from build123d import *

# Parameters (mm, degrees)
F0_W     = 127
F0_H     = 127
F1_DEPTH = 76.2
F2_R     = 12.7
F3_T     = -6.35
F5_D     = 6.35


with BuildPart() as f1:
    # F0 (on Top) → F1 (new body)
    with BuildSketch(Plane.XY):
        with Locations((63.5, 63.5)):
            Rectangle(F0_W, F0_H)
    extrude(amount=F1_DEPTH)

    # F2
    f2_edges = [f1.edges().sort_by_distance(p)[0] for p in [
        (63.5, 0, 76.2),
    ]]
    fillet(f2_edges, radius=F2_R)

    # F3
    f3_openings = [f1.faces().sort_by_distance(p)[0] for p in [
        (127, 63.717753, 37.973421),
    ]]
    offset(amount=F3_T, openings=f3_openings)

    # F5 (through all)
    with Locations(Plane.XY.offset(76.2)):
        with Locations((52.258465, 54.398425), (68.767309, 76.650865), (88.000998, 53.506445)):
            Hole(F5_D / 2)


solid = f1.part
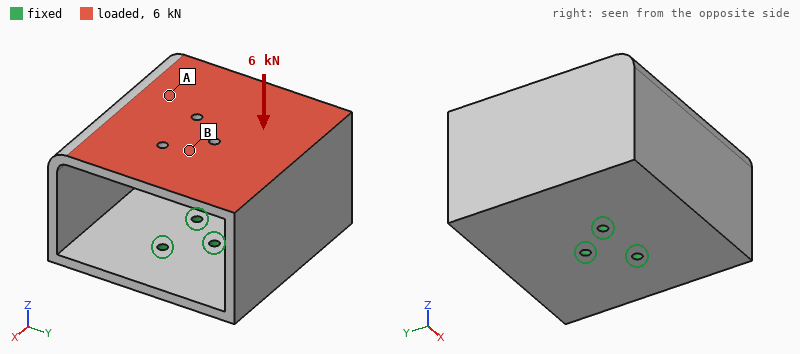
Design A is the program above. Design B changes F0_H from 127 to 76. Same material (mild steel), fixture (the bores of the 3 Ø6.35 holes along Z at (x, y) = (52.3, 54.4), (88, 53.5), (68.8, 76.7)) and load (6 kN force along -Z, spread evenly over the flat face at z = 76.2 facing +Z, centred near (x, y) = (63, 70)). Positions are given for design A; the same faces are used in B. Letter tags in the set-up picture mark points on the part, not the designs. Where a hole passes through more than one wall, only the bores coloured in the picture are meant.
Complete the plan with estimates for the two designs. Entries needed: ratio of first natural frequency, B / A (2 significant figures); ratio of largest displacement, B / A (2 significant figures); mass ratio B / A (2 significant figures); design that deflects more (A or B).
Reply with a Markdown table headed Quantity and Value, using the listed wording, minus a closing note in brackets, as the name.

| Quantity | Value |
|---|---|
| ratio of first natural frequency, B / A | 1.7 |
| ratio of largest displacement, B / A | 0.23 |
| mass ratio B / A | 0.71 |
| design that deflects more | A |
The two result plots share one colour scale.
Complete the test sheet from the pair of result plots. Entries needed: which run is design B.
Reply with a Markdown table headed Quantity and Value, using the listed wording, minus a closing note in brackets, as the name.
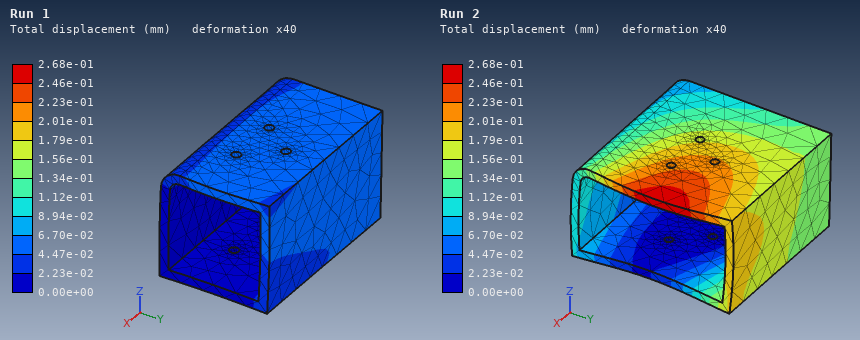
| Quantity | Value |
|---|---|
| which run is design B | Run 1 |
